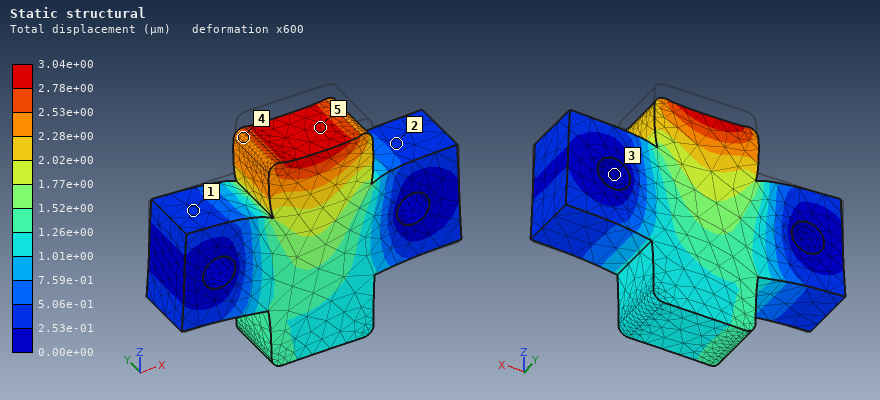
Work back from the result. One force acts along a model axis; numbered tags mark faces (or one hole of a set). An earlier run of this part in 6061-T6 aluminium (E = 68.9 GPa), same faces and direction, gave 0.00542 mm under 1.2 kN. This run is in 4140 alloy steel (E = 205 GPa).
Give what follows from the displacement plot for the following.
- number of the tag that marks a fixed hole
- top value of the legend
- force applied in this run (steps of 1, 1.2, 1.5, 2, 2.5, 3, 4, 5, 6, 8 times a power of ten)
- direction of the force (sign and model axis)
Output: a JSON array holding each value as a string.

["3", "3.04e+00 µm", "2 kN", "-Z"]
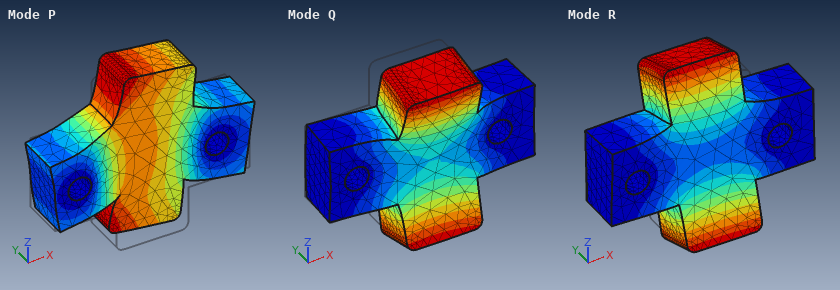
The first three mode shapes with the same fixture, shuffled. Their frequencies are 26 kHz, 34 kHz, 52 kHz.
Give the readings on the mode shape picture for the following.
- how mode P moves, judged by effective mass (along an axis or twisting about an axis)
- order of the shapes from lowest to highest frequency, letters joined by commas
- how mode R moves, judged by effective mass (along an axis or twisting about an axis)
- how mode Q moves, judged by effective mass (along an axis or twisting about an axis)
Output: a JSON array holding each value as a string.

["along Z", "R, Q, P", "twisting about X", "along Y"]
